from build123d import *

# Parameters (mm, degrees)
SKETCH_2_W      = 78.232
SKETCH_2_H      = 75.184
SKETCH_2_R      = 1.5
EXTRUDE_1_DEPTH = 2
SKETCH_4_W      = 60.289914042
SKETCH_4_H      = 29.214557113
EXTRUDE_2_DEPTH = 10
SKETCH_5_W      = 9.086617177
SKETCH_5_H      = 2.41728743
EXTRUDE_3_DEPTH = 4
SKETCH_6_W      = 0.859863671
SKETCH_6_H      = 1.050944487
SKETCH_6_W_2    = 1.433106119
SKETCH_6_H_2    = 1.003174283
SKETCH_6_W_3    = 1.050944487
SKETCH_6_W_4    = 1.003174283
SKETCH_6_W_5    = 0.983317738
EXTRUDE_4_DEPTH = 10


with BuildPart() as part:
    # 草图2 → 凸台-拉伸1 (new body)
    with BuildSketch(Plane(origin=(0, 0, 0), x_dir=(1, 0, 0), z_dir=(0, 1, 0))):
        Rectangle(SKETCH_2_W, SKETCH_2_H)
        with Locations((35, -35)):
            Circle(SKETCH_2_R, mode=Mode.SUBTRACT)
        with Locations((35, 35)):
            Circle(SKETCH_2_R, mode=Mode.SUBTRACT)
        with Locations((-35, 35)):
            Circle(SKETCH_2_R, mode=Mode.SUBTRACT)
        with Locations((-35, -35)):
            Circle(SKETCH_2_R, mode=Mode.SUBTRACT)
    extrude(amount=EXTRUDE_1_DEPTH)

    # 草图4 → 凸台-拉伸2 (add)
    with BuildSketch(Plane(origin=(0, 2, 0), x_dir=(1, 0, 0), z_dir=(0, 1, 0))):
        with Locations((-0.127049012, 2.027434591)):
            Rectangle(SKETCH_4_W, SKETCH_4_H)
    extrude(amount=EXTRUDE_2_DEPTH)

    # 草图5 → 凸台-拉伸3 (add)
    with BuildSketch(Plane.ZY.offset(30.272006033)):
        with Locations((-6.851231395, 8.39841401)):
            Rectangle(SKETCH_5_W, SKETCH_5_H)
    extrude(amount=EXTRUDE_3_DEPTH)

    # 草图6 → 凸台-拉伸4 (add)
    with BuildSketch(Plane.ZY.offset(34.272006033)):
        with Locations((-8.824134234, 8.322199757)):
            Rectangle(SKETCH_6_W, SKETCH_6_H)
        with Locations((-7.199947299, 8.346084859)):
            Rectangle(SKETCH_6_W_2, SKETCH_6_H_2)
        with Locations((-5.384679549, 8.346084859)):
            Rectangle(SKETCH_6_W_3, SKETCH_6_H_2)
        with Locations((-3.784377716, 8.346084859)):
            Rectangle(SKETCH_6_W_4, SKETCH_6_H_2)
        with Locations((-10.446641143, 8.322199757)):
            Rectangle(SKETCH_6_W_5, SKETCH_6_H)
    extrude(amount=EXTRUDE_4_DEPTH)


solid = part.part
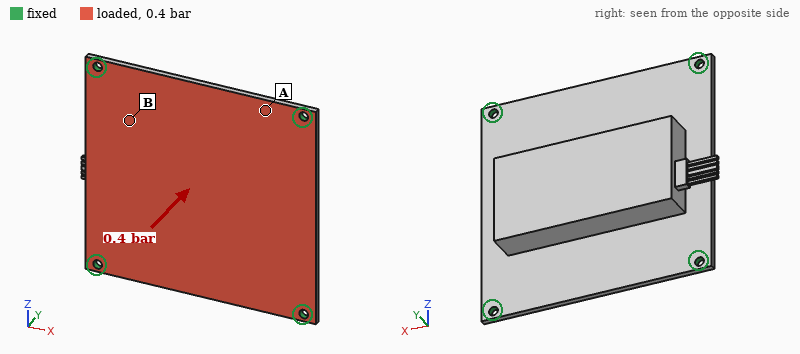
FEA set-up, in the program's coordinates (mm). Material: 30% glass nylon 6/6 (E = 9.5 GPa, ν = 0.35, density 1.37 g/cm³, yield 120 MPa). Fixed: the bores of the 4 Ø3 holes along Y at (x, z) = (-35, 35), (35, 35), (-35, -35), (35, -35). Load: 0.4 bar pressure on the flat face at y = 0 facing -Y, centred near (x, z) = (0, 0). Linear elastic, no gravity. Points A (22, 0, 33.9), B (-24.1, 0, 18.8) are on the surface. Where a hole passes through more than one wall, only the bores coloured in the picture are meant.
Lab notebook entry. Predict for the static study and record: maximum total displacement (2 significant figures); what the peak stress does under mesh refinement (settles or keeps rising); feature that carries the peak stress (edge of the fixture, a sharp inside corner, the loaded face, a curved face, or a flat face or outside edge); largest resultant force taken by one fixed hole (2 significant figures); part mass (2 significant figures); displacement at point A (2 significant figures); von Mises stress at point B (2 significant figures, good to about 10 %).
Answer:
0.42 mm
keeps rising
edge of the fixture
62 N
40 g
0.17 mm
16 MPa
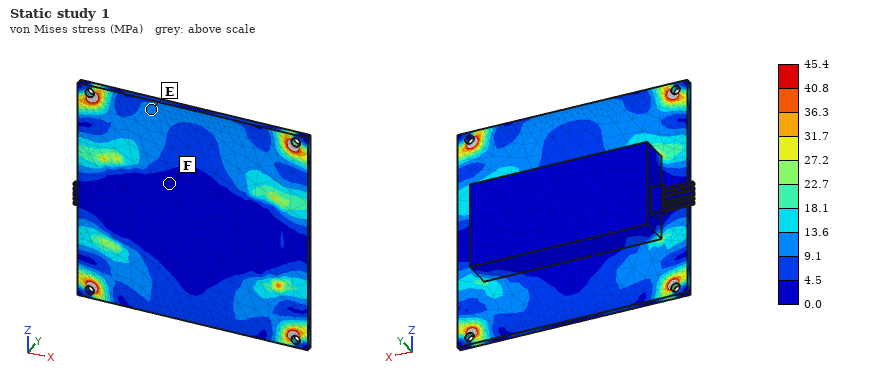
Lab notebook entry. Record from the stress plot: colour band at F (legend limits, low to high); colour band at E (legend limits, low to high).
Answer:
0.0 to 4.5 MPa
9.1 to 13.6 MPa
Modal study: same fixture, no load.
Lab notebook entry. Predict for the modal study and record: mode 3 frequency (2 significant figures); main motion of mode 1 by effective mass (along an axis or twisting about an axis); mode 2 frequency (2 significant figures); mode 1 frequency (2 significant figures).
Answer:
1300 Hz
along Y
990 Hz
600 Hz
